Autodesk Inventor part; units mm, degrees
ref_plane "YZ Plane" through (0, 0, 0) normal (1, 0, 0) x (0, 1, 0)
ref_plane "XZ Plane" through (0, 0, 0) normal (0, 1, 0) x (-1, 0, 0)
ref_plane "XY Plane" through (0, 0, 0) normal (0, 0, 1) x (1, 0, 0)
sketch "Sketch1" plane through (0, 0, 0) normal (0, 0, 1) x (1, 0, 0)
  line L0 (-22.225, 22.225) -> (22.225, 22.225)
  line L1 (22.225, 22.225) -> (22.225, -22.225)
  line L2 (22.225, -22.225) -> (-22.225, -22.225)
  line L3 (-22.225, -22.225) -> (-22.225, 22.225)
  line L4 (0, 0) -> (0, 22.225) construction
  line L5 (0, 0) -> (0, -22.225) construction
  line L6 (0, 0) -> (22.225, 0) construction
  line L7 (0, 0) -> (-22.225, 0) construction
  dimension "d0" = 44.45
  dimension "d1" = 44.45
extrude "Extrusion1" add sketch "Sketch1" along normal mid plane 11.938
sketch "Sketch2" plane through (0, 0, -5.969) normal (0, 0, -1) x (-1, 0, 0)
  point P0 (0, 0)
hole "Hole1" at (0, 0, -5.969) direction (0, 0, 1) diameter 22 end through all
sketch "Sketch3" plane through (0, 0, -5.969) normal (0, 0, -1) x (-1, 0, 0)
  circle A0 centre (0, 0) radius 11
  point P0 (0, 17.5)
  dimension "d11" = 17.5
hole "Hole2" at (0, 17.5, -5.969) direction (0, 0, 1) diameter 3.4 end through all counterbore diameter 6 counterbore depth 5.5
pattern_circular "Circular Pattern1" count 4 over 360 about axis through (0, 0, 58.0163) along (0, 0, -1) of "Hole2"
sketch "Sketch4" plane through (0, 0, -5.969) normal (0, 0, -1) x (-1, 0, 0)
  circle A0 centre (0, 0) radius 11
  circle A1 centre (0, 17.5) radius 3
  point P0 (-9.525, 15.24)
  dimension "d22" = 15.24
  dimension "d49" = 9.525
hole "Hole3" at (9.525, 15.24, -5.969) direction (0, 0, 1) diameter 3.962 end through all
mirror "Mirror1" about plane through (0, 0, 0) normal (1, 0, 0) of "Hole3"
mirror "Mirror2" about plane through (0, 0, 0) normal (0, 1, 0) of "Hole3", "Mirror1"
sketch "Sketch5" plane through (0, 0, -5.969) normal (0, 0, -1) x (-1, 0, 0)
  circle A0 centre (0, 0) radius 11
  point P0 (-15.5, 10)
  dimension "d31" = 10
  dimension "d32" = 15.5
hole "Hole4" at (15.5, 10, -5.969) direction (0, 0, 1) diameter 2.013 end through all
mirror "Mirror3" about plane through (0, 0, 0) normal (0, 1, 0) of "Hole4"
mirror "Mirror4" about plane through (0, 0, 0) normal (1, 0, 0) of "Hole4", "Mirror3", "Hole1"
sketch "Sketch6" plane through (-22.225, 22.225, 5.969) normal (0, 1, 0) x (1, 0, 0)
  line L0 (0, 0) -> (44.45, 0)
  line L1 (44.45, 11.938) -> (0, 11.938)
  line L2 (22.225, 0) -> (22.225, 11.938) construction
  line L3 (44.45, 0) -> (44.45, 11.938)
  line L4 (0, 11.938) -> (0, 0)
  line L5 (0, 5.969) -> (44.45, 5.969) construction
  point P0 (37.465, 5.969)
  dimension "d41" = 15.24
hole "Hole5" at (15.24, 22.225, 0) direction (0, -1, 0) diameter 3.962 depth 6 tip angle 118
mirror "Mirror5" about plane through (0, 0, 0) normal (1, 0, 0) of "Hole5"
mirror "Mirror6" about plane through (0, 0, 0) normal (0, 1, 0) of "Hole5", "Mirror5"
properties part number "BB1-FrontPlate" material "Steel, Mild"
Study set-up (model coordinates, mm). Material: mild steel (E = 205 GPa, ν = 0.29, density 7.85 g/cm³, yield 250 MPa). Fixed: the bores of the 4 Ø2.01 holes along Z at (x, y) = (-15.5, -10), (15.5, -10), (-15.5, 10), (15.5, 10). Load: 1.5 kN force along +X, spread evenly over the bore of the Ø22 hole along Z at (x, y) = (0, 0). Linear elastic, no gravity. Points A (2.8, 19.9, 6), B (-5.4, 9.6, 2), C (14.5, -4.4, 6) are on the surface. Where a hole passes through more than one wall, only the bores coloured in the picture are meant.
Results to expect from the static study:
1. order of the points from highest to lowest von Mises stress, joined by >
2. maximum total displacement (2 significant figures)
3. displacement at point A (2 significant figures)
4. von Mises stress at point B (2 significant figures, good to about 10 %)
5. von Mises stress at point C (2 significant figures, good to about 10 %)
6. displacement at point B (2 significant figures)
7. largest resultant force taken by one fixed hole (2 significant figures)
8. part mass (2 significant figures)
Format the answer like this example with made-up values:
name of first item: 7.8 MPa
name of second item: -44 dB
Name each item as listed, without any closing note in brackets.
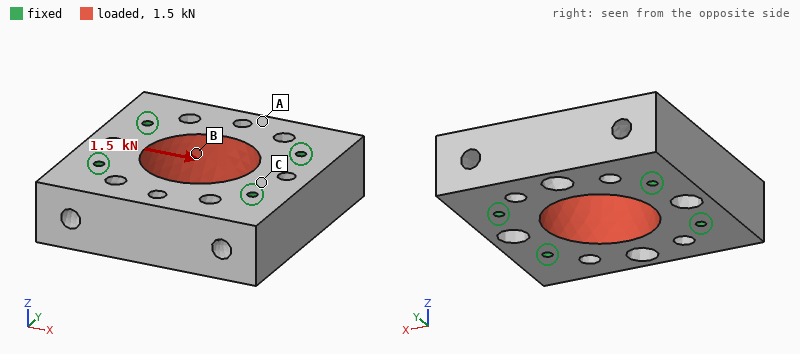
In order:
order of the points from highest to lowest von Mises stress, joined by >: B > C > A
maximum total displacement: 0.22 µm
displacement at point A: 0.092 µm
von Mises stress at point B: 3.2 MPa
von Mises stress at point C: 1.6 MPa
displacement at point B: 0.15 µm
largest resultant force taken by one fixed hole: 380 N
part mass: 130 g
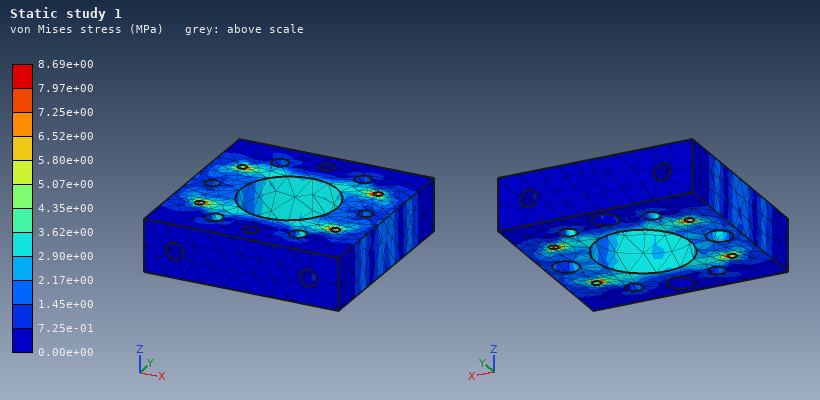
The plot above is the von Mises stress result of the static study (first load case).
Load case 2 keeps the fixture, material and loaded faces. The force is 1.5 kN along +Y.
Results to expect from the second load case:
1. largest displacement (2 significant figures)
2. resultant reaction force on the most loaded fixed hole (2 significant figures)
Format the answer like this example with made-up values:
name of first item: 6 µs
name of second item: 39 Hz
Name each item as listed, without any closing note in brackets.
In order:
largest displacement: 0.51 µm
resultant reaction force on the most loaded fixed hole: 380 N
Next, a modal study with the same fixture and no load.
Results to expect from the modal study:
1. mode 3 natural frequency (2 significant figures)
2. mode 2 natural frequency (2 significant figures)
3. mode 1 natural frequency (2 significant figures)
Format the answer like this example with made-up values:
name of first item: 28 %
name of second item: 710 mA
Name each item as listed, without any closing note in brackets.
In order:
mode 3 natural frequency: 35 kHz
mode 2 natural frequency: 25 kHz
mode 1 natural frequency: 25 kHz
